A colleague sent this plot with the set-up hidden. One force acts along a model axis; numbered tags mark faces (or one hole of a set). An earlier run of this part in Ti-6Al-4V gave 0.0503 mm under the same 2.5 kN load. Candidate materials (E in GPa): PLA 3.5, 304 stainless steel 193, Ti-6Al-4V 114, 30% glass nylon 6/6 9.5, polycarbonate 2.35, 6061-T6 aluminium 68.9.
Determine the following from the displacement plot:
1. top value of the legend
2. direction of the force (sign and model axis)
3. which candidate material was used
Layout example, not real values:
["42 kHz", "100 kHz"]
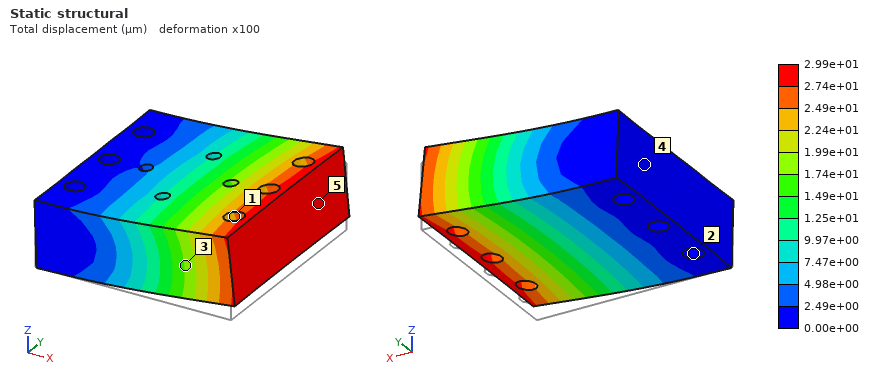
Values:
["2.99e+01 µm", "+Z", "304 stainless steel"]
